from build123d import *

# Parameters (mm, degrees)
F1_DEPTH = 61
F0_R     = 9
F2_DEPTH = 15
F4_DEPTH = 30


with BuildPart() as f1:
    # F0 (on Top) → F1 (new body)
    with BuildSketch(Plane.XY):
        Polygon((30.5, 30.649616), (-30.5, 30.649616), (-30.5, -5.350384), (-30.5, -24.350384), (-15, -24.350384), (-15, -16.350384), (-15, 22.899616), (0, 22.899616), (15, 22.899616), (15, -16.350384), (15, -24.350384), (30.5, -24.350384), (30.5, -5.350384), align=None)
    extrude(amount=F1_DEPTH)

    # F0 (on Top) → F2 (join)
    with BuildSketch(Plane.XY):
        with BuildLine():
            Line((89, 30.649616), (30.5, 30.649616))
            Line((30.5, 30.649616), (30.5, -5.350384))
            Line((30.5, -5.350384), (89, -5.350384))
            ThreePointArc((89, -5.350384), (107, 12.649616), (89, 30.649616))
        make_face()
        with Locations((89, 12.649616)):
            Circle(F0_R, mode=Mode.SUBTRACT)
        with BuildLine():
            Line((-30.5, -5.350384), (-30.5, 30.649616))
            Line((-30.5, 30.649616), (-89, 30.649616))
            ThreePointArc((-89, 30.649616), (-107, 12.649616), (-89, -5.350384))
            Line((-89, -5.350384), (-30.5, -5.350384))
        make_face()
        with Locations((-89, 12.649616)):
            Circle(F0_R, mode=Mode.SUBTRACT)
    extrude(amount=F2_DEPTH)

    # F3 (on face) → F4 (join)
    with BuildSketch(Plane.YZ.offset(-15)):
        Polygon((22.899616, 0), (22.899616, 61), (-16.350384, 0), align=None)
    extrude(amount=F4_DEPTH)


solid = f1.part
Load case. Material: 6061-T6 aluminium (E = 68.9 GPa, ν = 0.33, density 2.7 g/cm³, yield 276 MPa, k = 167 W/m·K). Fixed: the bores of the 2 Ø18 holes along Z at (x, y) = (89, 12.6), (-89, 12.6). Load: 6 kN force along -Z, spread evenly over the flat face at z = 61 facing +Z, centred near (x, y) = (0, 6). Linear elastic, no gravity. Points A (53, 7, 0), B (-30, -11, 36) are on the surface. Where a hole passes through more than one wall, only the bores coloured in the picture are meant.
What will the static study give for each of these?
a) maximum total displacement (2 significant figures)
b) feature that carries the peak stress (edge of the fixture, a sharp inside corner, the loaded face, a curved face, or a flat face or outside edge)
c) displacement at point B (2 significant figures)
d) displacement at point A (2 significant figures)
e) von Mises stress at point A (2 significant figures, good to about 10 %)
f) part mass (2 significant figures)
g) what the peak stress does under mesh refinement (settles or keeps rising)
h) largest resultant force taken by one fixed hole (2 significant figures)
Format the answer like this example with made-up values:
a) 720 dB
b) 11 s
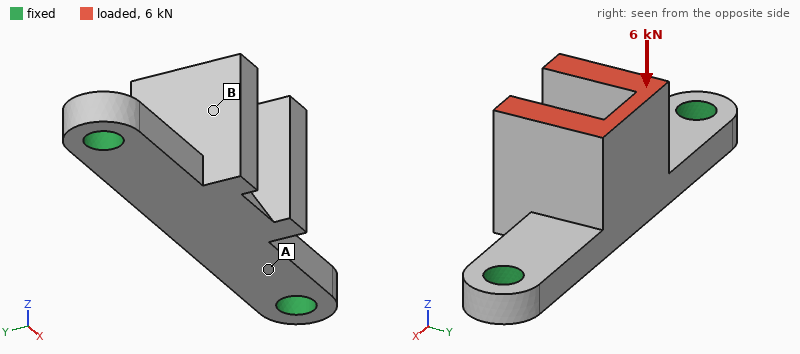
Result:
a) 0.16 mm
b) edge of the fixture
c) 0.13 mm
d) 0.051 mm
e) 17 MPa
f) 610 g
g) keeps rising
h) 3.3 kN
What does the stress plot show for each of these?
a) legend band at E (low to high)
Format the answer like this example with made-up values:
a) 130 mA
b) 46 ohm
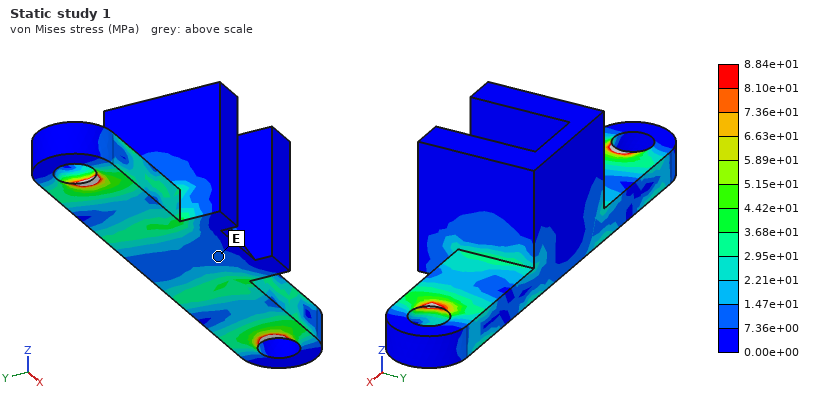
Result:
a) 7.36e+00 to 1.47e+01 MPa
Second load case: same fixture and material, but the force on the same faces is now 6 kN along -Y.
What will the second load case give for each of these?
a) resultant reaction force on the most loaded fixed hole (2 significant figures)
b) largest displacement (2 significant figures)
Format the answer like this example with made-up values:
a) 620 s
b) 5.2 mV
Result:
a) 3.0 kN
b) 0.74 mm
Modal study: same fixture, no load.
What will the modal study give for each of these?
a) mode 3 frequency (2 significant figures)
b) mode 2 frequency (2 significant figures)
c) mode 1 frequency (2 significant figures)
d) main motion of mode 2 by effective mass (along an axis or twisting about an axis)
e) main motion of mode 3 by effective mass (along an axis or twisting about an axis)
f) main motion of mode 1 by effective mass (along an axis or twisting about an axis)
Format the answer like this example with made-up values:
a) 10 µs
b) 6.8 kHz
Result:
a) 3200 Hz
b) 1900 Hz
c) 1300 Hz
d) along Z
e) along X
f) along Y
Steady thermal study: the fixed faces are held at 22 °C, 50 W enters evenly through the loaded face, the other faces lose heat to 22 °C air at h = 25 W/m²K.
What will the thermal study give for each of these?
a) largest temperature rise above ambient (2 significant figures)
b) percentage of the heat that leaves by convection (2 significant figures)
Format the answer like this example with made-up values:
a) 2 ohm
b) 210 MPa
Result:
a) 20 K
b) 19 %
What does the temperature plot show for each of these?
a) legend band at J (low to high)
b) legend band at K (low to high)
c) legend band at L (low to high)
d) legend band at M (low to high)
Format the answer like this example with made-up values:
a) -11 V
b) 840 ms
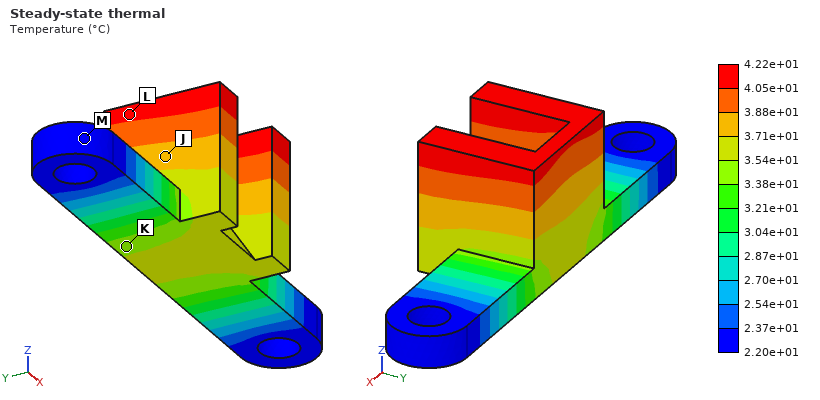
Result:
a) 3.71e+01 to 3.88e+01 °C
b) 3.38e+01 to 3.54e+01 °C
c) 4.05e+01 to 4.22e+01 °C
d) 2.20e+01 to 2.37e+01 °C
